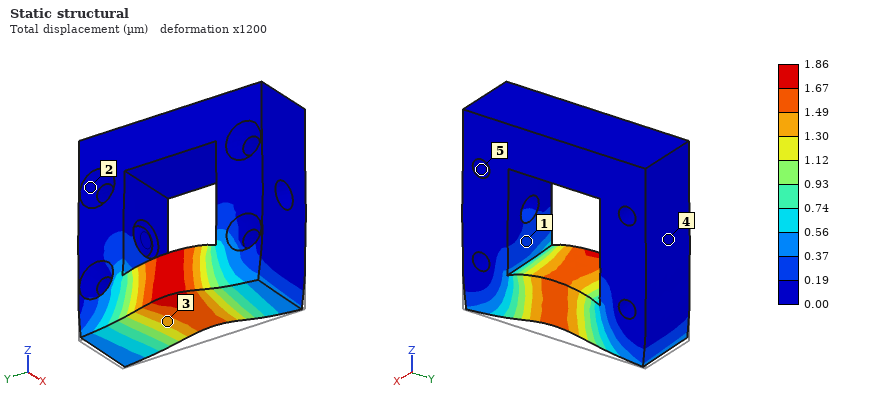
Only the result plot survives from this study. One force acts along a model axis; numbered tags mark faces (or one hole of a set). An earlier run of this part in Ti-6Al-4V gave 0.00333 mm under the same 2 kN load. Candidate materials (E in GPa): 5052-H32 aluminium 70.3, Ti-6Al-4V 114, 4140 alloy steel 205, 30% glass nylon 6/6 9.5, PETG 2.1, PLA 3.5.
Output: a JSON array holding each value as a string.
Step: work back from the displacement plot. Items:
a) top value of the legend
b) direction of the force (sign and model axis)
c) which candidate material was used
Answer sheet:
["1.86 µm", "+Z", "4140 alloy steel"]
